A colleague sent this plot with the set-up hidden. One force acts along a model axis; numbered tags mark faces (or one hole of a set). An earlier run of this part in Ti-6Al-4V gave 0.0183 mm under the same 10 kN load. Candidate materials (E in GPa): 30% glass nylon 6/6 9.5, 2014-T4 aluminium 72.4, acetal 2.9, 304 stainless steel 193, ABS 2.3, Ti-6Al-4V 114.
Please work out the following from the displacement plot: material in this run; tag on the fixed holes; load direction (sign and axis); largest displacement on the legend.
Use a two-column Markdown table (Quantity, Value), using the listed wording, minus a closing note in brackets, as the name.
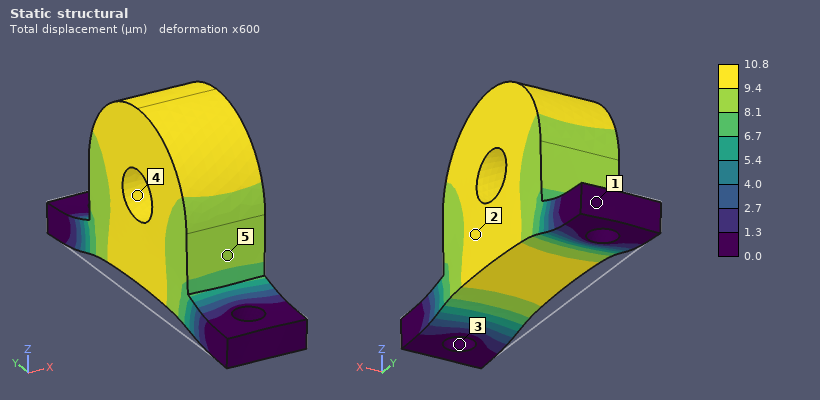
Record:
| Quantity | Value |
|---|---|
| material in this run | 304 stainless steel |
| tag on the fixed holes | 3 |
| load direction | +Z |
| largest displacement on the legend | 10.8 µm |
